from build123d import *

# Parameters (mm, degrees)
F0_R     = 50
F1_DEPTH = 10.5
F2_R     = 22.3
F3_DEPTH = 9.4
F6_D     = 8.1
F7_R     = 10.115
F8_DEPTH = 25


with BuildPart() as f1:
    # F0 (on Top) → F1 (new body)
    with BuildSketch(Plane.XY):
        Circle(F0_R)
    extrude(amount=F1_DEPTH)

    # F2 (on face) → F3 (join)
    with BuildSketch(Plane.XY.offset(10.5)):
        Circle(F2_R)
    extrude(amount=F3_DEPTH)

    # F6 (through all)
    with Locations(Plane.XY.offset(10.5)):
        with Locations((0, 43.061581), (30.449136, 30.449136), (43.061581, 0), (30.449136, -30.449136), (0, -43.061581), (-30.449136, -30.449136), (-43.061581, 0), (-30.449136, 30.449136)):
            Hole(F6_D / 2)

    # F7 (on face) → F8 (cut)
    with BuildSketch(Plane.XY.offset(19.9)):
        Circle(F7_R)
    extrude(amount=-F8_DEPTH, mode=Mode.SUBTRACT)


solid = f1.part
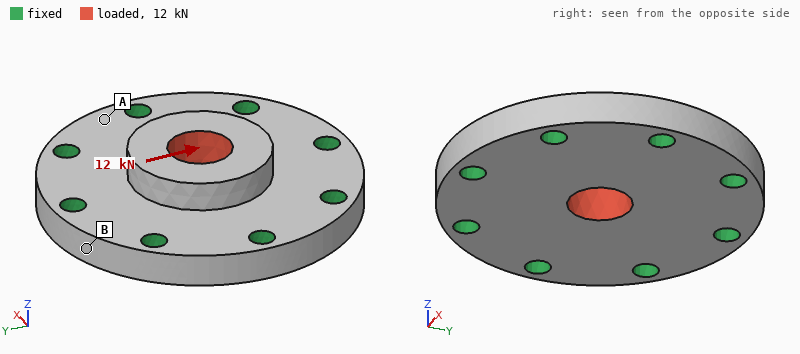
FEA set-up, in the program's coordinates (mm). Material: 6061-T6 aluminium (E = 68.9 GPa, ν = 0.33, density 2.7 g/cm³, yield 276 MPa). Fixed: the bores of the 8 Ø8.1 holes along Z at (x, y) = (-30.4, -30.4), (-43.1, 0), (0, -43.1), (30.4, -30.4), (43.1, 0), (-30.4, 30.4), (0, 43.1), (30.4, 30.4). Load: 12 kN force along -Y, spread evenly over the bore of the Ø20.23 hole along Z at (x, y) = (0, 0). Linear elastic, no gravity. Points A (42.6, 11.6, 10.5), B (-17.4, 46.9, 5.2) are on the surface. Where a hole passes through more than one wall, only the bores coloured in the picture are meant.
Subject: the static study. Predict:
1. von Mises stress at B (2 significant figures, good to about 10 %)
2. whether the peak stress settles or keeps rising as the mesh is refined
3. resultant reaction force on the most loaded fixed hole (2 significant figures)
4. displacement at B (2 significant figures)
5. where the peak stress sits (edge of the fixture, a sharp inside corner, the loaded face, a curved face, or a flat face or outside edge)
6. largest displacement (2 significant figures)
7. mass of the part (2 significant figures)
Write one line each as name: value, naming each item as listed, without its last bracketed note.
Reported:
von Mises stress at B: 5.3 MPa
whether the peak stress settles or keeps rising as the mesh is refined: keeps rising
resultant reaction force on the most loaded fixed hole: 2.5 kN
displacement at B: 1.4 µm
where the peak stress sits: edge of the fixture
largest displacement: 8.7 µm
mass of the part: 230 g
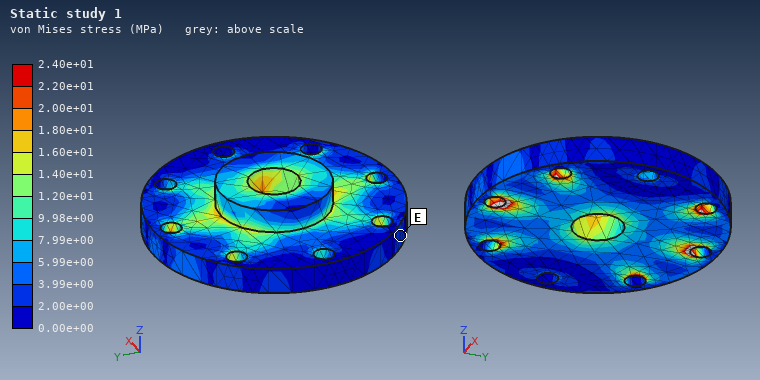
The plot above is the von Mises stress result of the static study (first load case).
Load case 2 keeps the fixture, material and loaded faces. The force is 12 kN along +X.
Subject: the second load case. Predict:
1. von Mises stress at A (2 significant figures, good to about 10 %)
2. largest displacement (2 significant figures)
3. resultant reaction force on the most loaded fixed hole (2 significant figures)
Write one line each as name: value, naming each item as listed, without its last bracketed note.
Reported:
von Mises stress at A: 2.7 MPa
largest displacement: 8.7 µm
resultant reaction force on the most loaded fixed hole: 2.5 kN
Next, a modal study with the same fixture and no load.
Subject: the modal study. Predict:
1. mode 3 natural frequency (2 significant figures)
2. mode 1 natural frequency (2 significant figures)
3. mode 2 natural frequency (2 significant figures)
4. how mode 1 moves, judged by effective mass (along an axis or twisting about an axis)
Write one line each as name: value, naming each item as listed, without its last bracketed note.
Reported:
mode 3 natural frequency: 20 kHz
mode 1 natural frequency: 13 kHz
mode 2 natural frequency: 20 kHz
how mode 1 moves, judged by effective mass: along Z
